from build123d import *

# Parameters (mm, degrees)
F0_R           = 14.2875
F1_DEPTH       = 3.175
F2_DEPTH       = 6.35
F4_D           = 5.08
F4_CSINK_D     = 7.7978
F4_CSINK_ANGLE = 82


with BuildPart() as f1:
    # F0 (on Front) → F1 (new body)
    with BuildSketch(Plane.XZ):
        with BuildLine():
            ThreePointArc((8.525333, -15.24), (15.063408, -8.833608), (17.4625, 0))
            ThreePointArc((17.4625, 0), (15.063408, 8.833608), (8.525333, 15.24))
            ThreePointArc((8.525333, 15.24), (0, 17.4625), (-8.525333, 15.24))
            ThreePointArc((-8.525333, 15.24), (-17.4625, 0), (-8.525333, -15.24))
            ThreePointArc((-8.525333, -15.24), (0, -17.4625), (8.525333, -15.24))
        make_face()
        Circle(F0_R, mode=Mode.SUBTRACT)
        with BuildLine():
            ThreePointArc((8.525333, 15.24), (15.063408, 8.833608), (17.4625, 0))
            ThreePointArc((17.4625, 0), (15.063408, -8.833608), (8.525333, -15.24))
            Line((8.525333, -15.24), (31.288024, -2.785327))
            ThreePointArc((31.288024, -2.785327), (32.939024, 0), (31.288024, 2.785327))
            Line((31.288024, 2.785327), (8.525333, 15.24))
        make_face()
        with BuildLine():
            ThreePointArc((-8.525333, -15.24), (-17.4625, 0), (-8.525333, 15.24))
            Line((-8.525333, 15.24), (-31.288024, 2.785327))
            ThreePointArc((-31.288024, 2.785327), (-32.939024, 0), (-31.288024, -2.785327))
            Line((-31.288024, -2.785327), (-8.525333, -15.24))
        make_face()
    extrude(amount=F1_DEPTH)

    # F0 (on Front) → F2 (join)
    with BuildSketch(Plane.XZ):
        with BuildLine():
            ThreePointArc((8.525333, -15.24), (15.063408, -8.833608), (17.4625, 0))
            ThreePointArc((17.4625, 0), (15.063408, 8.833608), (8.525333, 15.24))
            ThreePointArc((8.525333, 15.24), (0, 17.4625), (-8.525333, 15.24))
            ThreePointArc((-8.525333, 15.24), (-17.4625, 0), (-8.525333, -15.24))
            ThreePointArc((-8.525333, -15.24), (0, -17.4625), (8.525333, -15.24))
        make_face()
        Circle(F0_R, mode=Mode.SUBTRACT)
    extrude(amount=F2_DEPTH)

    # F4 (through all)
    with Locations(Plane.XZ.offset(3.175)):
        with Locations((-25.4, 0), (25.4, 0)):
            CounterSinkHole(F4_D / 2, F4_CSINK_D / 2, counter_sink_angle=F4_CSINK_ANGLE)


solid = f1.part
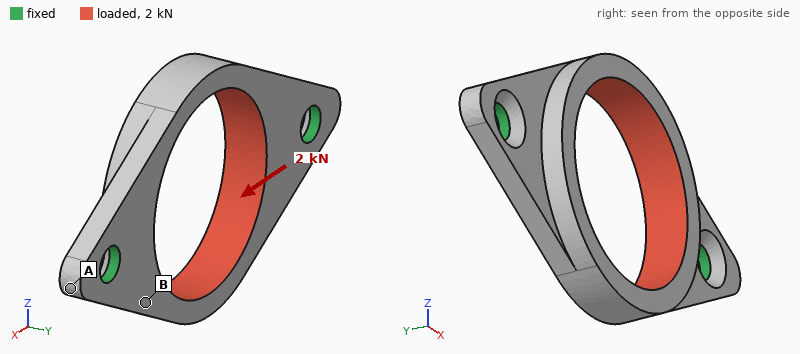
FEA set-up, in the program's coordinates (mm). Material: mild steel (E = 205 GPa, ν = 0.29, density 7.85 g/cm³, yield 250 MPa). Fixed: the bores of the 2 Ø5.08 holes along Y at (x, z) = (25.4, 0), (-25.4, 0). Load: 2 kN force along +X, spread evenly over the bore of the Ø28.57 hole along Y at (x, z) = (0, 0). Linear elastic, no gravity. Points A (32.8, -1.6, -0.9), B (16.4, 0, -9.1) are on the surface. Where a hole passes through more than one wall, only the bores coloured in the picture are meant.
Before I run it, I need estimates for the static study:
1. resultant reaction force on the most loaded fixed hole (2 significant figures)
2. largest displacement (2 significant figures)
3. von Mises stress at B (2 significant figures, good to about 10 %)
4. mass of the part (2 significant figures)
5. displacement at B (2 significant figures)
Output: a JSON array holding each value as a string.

["1.0 kN", "5.8 µm", "29 MPa", "26 g", "2.3 µm"]
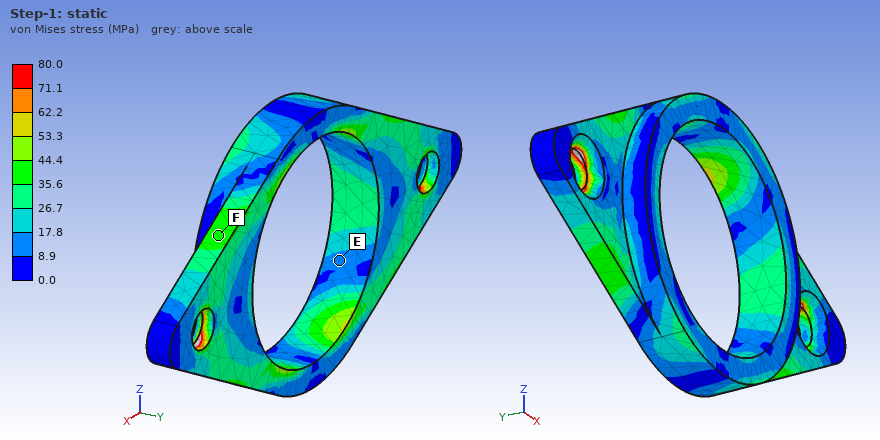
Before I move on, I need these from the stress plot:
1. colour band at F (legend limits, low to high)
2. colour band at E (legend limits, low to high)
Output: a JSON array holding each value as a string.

["35.6 to 44.4 MPa", "8.9 to 17.8 MPa"]
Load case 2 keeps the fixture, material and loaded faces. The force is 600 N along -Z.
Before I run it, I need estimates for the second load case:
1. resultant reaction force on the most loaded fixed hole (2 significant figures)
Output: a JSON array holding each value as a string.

["300 N"]
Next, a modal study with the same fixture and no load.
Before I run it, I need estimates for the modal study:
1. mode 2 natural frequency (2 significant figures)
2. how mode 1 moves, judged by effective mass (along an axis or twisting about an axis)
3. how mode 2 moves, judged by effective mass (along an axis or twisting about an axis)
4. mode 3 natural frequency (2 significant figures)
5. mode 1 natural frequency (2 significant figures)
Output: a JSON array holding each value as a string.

["6100 Hz", "twisting about X", "along Y", "14 kHz", "4800 Hz"]
